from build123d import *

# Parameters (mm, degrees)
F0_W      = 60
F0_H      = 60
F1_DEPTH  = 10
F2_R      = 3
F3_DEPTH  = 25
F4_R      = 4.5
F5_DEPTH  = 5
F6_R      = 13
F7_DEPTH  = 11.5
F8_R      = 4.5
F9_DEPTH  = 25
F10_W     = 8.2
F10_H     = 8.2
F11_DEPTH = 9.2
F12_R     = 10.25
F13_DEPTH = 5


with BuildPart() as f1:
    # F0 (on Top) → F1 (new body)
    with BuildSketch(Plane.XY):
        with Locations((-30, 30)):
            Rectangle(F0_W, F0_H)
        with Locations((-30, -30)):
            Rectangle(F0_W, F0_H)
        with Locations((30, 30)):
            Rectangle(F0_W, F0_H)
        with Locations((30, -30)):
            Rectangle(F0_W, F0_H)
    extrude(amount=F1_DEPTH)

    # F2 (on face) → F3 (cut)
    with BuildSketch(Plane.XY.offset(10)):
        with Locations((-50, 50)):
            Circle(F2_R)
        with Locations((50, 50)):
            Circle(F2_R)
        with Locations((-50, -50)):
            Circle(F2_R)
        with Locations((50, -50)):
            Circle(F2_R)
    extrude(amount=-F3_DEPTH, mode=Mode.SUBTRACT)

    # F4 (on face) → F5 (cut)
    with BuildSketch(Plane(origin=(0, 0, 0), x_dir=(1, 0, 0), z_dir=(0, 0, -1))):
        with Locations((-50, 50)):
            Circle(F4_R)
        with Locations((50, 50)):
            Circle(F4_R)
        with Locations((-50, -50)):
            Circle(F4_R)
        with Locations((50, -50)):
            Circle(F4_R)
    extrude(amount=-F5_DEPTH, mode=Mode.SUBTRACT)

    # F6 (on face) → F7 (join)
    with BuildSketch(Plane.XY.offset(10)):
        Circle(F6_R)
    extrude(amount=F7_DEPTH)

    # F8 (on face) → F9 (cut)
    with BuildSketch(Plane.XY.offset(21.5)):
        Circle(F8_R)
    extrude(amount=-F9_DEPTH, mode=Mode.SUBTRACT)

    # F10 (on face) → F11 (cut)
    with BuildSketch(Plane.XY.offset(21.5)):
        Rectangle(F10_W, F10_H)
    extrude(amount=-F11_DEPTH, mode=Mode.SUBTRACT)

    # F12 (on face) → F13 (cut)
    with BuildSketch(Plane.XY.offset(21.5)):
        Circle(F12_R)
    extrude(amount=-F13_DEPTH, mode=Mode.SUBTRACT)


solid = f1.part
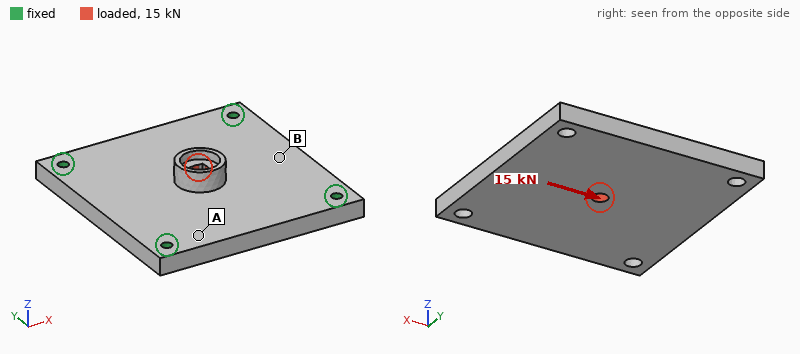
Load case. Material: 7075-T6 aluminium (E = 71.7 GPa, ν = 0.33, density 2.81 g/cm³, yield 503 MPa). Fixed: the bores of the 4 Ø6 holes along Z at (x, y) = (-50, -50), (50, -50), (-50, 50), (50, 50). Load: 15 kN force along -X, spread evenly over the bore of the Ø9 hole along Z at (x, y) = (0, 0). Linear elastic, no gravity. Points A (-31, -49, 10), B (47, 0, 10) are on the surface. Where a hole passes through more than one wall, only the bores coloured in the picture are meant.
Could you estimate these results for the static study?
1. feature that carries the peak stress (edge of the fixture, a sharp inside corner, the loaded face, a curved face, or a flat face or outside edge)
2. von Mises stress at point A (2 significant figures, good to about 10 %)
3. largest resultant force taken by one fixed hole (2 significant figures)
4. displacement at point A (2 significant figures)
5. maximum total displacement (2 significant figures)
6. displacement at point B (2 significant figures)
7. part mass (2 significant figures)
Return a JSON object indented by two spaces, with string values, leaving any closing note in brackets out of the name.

{
  "feature that carries the peak stress": "edge of the fixture",
  "von Mises stress at point A": "20 MPa",
  "largest resultant force taken by one fixed hole": "4.0 kN",
  "displacement at point A": "7.5 µm",
  "maximum total displacement": "36 µm",
  "displacement at point B": "22 µm",
  "part mass": "410 g"
}
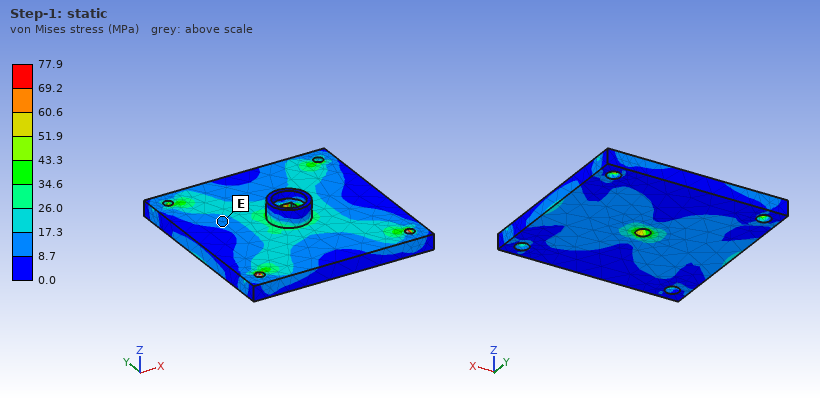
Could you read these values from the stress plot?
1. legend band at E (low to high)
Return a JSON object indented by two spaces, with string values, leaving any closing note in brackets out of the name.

{
  "legend band at E": "8.7 to 17.3 MPa"
}
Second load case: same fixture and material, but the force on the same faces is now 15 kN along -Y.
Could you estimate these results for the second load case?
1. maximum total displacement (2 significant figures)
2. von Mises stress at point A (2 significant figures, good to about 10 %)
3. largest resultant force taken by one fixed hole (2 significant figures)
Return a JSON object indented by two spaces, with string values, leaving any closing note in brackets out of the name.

{
  "maximum total displacement": "36 µm",
  "von Mises stress at point A": "13 MPa",
  "largest resultant force taken by one fixed hole": "4.0 kN"
}
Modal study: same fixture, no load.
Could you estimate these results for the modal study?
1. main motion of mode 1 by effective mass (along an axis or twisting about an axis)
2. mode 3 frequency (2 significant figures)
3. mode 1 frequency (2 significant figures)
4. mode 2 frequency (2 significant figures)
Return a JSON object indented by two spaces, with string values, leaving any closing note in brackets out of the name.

{
  "main motion of mode 1 by effective mass": "along Z",
  "mode 3 frequency": "4500 Hz",
  "mode 1 frequency": "2600 Hz",
  "mode 2 frequency": "4500 Hz"
}
